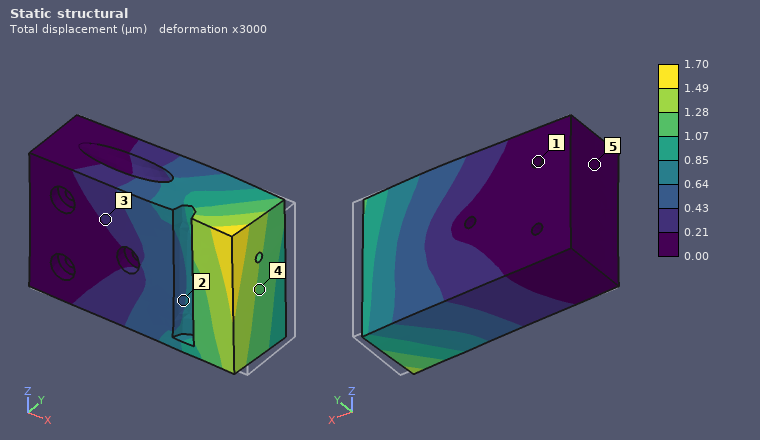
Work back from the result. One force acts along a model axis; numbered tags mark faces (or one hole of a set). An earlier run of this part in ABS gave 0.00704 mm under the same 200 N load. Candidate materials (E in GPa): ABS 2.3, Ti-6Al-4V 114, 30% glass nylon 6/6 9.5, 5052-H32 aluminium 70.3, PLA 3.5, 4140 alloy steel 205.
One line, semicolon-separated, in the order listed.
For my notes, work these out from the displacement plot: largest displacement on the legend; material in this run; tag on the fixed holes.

1.70 µm; 30% glass nylon 6/6; 1
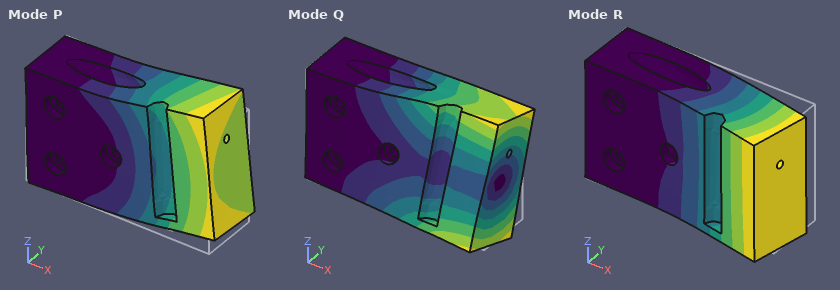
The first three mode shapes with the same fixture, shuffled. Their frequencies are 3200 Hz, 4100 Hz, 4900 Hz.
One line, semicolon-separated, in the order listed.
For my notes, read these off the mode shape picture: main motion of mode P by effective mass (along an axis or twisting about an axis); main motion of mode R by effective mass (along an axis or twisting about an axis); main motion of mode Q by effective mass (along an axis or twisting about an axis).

along Z; along Y; twisting about X
